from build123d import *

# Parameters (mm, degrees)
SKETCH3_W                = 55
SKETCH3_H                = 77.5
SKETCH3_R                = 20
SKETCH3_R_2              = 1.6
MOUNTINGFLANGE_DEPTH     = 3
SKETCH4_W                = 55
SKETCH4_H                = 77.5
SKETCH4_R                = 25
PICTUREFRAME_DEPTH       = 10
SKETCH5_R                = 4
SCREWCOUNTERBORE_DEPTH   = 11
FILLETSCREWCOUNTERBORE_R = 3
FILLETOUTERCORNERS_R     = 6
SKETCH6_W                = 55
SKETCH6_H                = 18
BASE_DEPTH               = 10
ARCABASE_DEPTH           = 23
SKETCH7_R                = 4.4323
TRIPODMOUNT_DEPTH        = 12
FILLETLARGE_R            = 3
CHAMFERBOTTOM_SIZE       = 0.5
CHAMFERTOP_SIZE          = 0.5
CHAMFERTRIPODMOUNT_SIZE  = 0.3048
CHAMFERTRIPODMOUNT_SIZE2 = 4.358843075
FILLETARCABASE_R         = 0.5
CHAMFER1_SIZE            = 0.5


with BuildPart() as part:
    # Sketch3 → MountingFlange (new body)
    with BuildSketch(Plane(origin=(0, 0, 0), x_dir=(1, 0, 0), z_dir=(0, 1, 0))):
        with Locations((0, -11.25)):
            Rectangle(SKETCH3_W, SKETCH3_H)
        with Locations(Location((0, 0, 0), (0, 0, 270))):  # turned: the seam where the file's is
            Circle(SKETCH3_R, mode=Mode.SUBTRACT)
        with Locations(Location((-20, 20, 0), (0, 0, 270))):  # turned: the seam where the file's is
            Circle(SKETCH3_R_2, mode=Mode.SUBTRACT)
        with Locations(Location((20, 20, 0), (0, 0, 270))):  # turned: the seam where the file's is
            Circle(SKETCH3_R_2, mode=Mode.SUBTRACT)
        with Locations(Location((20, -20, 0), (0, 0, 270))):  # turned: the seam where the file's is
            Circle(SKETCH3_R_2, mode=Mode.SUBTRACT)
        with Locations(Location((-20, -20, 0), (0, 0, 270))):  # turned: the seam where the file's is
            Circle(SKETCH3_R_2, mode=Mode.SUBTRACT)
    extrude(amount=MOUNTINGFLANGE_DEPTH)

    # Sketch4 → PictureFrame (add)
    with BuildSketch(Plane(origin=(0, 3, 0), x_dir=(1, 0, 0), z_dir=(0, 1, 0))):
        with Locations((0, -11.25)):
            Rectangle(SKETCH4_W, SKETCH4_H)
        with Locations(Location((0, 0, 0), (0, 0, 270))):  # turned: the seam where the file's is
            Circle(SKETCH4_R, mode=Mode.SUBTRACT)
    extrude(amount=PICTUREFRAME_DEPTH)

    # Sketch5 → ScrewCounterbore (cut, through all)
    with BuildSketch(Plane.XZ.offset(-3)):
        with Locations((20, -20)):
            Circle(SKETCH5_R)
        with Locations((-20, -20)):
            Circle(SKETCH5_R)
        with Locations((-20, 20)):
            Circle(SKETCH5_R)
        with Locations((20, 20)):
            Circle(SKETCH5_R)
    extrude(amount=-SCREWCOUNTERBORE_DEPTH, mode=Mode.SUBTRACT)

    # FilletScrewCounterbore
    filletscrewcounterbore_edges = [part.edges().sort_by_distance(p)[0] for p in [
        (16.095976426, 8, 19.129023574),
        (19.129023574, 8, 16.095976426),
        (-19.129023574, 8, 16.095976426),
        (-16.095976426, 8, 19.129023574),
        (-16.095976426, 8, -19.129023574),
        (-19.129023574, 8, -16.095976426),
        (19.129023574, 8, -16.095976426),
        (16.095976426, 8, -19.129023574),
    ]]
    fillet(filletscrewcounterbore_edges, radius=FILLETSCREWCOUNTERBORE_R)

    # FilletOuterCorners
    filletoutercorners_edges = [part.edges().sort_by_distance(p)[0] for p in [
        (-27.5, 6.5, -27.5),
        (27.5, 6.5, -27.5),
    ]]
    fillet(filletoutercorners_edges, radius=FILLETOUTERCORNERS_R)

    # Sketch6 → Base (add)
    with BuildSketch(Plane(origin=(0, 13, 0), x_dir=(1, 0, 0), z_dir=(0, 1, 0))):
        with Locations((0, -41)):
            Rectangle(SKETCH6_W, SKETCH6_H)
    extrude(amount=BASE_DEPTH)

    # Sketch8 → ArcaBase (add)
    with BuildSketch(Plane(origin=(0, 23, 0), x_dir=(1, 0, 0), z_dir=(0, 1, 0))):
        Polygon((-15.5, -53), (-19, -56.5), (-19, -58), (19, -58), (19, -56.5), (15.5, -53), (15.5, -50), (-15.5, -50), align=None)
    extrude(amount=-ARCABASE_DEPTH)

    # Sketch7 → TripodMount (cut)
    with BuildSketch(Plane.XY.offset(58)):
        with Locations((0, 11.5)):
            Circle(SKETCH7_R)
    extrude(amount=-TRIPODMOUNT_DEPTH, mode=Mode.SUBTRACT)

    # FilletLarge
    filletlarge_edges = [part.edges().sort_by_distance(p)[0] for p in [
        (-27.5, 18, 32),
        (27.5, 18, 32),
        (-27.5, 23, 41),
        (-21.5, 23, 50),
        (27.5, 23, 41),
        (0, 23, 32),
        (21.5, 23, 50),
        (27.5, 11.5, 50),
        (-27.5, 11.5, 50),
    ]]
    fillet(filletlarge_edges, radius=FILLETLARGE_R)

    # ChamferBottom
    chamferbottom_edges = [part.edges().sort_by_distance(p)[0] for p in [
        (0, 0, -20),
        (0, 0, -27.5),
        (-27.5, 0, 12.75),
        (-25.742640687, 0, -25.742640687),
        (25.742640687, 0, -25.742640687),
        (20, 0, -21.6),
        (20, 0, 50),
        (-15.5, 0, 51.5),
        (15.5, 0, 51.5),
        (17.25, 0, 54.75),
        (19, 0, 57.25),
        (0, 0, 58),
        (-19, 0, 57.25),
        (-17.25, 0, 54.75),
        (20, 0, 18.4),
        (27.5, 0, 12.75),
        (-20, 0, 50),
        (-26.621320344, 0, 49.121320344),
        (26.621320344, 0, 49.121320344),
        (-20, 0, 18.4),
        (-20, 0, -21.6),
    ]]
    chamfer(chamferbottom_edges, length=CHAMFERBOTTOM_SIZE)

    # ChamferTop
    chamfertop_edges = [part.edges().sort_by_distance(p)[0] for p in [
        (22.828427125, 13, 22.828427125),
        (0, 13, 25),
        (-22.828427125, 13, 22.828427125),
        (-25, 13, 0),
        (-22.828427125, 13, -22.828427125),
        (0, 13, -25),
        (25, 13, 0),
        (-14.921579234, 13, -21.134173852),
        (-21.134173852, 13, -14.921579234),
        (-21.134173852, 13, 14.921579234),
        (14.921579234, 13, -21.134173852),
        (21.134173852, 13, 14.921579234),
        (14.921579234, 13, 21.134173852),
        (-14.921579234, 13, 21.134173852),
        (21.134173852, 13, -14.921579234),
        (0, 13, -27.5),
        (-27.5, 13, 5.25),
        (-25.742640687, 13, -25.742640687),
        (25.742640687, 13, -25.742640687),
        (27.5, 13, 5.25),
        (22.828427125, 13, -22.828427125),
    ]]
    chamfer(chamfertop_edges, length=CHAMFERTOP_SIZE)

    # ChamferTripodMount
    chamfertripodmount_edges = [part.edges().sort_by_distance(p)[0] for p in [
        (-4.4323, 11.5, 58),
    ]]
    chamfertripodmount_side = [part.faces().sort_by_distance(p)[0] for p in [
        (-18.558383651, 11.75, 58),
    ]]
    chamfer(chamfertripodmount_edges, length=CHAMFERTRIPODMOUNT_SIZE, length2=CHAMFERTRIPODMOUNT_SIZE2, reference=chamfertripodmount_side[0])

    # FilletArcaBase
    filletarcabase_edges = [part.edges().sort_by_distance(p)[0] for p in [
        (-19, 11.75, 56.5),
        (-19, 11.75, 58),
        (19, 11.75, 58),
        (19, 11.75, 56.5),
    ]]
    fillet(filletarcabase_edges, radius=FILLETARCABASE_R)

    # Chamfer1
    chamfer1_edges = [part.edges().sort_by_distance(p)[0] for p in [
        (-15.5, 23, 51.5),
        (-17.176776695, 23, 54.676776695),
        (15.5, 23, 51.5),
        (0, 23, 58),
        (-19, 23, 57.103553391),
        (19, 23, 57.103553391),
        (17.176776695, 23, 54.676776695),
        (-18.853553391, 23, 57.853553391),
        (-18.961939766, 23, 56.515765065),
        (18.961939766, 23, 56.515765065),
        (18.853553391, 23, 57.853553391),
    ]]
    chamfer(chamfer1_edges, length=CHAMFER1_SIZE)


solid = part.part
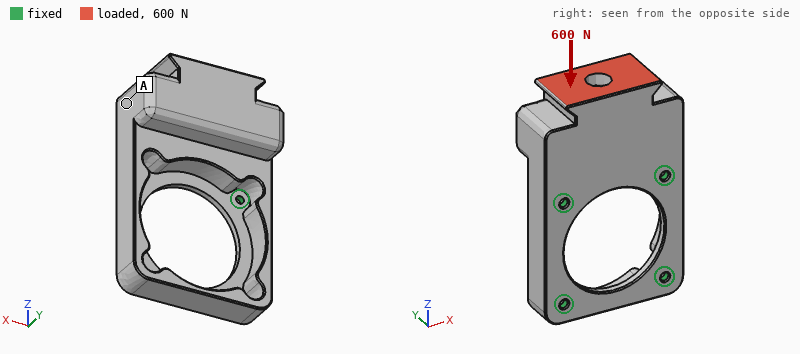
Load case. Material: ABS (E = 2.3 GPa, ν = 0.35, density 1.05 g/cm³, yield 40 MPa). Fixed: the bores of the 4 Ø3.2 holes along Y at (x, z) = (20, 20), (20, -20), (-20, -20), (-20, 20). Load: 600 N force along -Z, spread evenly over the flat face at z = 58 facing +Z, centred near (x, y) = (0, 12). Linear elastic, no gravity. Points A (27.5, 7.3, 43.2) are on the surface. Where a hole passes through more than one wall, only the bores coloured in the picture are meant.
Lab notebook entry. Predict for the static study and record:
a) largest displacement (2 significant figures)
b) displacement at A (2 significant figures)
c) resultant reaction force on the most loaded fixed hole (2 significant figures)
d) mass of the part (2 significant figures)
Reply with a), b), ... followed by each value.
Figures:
a) 0.90 mm
b) 0.46 mm
c) 200 N
d) 47 g
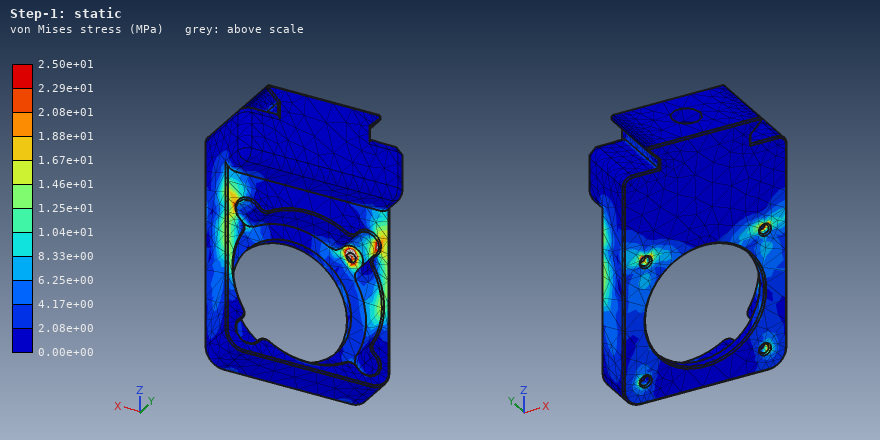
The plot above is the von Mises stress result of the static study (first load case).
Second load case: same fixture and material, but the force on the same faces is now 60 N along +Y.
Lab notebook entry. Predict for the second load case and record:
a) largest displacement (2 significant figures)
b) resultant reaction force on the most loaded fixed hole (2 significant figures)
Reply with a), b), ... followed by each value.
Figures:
a) 0.37 mm
b) 70 N
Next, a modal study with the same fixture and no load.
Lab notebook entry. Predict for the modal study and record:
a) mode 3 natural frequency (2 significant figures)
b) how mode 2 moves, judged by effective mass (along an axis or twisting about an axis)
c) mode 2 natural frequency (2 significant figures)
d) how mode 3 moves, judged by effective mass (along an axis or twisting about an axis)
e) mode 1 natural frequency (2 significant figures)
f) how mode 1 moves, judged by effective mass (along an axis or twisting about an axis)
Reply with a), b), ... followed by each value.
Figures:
a) 2400 Hz
b) along X
c) 1900 Hz
d) along X
e) 560 Hz
f) along Y
